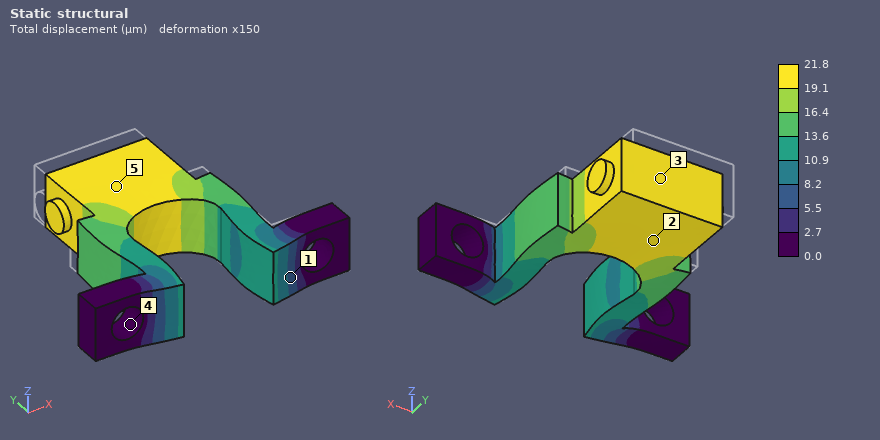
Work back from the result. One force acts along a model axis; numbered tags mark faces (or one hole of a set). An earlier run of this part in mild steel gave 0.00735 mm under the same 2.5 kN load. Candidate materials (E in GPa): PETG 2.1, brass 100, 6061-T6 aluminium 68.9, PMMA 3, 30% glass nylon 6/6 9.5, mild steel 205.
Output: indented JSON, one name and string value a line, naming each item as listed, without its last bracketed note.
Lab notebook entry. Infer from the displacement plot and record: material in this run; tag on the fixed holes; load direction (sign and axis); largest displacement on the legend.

{
  "material in this run": "6061-T6 aluminium",
  "tag on the fixed holes": "4",
  "load direction": "-Y",
  "largest displacement on the legend": "21.8 µm"
}
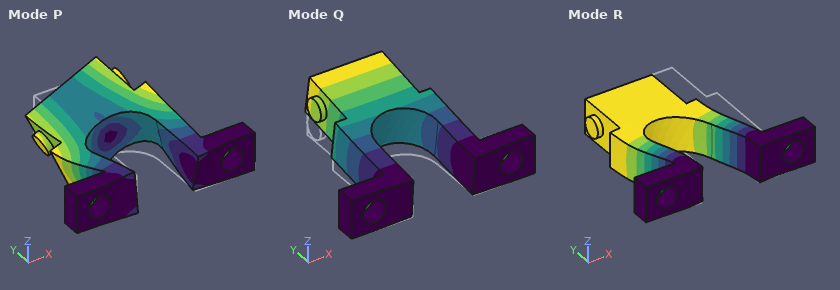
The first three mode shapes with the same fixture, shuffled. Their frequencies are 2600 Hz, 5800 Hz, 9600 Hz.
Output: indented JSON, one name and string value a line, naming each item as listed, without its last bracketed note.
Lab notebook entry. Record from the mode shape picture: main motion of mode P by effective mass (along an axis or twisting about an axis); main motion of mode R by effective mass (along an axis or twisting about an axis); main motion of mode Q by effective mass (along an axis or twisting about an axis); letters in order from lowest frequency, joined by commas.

{
  "main motion of mode P by effective mass": "twisting about Y",
  "main motion of mode R by effective mass": "along X",
  "main motion of mode Q by effective mass": "along Z",
  "letters in order from lowest frequency, joined by commas": "Q, R, P"
}
